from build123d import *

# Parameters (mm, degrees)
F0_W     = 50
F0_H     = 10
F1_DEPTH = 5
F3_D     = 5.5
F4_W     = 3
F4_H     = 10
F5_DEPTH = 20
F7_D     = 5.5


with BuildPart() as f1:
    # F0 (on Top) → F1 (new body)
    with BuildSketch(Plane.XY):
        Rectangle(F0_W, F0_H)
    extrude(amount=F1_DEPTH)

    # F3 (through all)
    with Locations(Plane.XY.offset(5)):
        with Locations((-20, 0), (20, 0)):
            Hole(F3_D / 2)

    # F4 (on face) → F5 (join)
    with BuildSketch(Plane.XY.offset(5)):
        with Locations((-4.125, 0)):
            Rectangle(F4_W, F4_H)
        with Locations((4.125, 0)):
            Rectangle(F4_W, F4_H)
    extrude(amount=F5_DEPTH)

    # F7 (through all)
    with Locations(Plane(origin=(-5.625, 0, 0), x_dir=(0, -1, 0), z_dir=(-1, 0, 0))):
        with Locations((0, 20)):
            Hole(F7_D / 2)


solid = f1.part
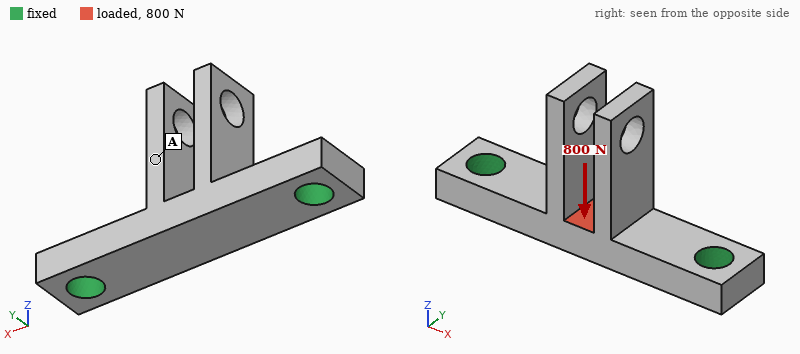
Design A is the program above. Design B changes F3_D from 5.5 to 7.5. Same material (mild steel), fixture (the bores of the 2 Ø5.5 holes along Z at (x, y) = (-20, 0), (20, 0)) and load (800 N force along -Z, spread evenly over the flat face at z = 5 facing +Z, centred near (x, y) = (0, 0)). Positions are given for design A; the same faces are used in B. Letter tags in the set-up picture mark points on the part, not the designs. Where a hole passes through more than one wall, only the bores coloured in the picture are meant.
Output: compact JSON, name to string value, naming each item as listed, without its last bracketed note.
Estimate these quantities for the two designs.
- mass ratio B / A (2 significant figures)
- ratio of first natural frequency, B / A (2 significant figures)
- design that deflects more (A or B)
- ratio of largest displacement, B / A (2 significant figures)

{"mass ratio B / A": "0.94", "ratio of first natural frequency, B / A": "1.0", "design that deflects more": "A", "ratio of largest displacement, B / A": "0.89"}
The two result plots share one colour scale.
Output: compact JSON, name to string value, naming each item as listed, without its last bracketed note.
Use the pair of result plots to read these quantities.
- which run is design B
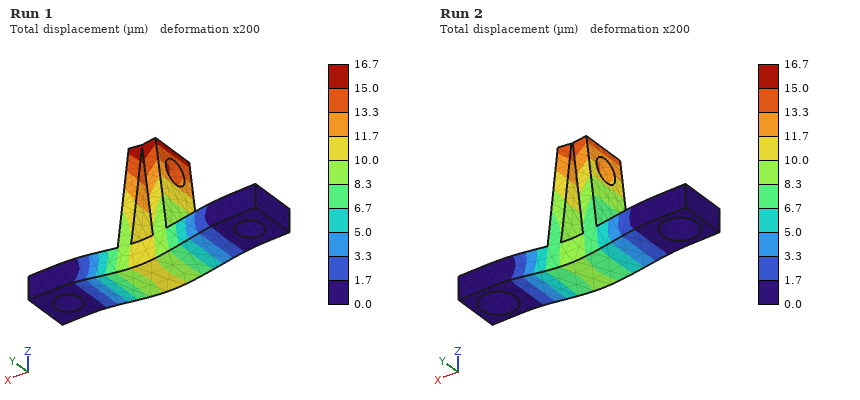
{"which run is design B": "Run 2"}
